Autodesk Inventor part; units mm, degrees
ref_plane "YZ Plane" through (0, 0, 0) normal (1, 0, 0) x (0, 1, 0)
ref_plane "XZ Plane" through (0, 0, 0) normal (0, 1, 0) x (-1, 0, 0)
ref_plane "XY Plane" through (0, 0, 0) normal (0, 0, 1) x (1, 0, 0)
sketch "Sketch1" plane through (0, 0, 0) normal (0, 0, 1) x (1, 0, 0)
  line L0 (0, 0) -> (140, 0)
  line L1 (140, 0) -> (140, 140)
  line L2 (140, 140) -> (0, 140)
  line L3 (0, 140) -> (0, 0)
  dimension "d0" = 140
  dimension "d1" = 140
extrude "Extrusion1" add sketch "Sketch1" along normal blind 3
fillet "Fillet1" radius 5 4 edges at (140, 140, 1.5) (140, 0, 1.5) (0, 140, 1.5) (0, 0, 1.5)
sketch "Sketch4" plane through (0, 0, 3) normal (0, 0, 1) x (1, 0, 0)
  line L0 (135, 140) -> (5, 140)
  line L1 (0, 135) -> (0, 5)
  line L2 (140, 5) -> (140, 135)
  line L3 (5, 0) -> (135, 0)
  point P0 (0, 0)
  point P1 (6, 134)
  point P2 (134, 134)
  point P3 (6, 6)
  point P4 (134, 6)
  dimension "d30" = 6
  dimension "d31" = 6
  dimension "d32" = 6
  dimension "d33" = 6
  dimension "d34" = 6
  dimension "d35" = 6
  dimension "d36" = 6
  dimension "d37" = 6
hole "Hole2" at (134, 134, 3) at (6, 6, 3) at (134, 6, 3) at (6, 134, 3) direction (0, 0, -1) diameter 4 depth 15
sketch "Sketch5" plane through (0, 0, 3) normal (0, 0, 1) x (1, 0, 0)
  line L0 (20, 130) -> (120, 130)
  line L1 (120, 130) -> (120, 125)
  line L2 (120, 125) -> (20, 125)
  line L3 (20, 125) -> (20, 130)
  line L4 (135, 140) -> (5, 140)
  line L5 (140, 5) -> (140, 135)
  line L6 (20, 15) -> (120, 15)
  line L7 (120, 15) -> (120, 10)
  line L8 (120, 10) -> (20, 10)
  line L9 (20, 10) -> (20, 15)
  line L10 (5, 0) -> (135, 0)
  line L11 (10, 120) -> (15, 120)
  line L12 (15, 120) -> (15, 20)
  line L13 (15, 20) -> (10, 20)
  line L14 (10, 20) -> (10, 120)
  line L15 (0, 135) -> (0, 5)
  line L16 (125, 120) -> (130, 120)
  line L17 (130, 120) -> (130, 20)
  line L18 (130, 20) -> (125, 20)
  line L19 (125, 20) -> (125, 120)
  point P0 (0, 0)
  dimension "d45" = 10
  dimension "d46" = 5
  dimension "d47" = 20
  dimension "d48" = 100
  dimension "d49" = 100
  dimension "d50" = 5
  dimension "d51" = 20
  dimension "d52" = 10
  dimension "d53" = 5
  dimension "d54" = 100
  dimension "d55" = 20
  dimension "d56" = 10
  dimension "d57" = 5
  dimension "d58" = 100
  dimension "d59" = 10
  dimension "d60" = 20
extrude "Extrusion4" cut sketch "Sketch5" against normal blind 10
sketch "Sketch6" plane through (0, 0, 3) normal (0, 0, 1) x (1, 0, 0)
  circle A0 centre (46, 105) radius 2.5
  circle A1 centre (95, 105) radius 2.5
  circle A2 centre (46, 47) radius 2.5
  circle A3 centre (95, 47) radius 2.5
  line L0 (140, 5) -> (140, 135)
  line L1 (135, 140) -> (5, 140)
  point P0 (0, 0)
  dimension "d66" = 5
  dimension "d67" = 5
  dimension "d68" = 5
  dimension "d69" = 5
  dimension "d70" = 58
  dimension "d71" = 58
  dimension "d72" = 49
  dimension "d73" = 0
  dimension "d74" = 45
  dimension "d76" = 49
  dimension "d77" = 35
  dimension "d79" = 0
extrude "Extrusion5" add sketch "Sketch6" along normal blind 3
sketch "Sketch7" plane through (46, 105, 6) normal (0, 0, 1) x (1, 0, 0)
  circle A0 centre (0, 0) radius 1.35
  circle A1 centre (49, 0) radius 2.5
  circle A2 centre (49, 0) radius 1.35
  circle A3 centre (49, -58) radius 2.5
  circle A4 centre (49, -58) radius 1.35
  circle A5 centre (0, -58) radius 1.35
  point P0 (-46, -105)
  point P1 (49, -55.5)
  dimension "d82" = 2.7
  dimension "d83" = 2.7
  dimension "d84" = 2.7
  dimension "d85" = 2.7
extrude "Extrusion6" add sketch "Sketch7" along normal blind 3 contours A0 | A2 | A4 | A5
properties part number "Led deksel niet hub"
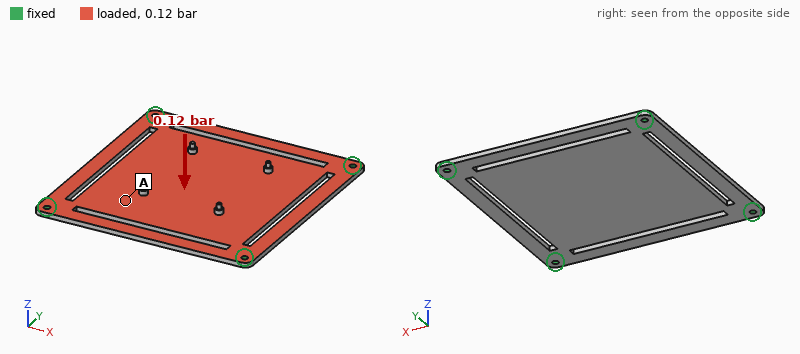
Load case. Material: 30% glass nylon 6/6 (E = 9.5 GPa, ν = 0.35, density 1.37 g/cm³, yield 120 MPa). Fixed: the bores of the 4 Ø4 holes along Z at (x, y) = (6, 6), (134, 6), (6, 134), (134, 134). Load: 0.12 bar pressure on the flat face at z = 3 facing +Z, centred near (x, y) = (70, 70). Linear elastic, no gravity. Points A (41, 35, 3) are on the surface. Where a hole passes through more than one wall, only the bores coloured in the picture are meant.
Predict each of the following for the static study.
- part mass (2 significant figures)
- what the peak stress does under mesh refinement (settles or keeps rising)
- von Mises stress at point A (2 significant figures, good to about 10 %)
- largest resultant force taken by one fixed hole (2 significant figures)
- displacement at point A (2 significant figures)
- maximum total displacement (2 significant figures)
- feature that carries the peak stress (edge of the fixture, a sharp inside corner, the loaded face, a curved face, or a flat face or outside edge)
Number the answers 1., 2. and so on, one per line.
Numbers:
1. 72 g
2. keeps rising
3. 6.8 MPa
4. 52 N
5. 0.94 mm
6. 1.3 mm
7. edge of the fixture
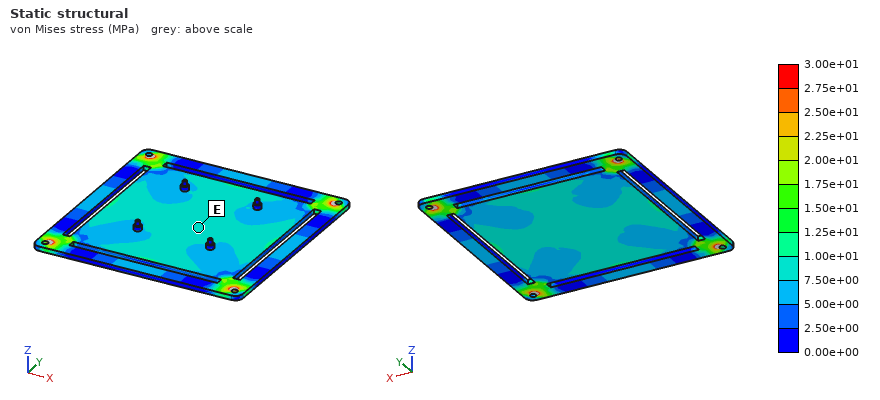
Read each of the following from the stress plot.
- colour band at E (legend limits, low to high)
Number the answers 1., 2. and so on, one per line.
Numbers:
1. 7.50e+00 to 1.00e+01 MPa
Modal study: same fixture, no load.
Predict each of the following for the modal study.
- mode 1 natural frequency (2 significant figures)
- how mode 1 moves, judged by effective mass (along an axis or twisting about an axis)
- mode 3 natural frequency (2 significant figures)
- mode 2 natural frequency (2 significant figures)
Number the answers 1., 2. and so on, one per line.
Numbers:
1. 270 Hz
2. along Z
3. 510 Hz
4. 510 Hz
